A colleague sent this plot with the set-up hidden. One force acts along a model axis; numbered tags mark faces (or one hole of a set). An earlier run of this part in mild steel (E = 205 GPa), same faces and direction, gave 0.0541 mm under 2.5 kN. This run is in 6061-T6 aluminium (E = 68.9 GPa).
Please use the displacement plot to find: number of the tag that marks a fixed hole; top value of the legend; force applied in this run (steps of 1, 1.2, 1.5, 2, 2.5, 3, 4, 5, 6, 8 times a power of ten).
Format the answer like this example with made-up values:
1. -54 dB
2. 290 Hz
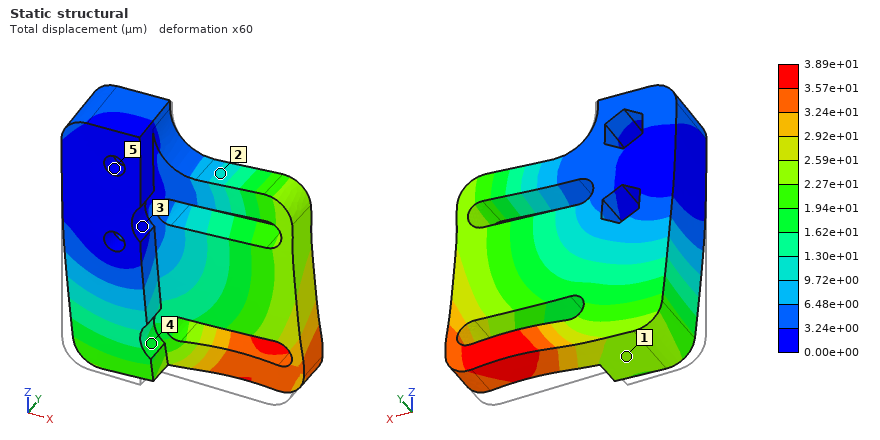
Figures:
1. 5
2. 3.89e+01 µm
3. 600 N
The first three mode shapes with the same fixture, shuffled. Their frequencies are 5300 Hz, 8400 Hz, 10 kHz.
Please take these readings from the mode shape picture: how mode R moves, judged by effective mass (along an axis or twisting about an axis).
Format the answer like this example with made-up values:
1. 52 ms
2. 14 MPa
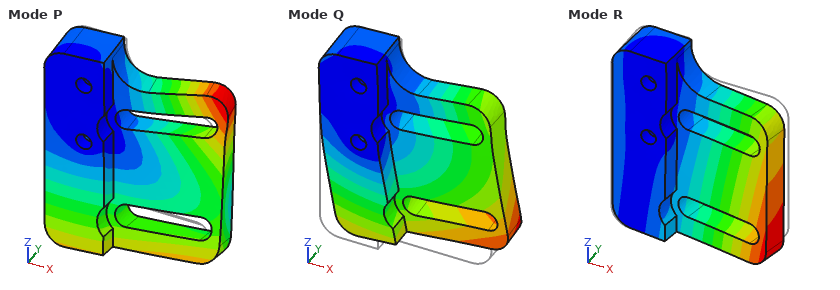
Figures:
1. along Y
